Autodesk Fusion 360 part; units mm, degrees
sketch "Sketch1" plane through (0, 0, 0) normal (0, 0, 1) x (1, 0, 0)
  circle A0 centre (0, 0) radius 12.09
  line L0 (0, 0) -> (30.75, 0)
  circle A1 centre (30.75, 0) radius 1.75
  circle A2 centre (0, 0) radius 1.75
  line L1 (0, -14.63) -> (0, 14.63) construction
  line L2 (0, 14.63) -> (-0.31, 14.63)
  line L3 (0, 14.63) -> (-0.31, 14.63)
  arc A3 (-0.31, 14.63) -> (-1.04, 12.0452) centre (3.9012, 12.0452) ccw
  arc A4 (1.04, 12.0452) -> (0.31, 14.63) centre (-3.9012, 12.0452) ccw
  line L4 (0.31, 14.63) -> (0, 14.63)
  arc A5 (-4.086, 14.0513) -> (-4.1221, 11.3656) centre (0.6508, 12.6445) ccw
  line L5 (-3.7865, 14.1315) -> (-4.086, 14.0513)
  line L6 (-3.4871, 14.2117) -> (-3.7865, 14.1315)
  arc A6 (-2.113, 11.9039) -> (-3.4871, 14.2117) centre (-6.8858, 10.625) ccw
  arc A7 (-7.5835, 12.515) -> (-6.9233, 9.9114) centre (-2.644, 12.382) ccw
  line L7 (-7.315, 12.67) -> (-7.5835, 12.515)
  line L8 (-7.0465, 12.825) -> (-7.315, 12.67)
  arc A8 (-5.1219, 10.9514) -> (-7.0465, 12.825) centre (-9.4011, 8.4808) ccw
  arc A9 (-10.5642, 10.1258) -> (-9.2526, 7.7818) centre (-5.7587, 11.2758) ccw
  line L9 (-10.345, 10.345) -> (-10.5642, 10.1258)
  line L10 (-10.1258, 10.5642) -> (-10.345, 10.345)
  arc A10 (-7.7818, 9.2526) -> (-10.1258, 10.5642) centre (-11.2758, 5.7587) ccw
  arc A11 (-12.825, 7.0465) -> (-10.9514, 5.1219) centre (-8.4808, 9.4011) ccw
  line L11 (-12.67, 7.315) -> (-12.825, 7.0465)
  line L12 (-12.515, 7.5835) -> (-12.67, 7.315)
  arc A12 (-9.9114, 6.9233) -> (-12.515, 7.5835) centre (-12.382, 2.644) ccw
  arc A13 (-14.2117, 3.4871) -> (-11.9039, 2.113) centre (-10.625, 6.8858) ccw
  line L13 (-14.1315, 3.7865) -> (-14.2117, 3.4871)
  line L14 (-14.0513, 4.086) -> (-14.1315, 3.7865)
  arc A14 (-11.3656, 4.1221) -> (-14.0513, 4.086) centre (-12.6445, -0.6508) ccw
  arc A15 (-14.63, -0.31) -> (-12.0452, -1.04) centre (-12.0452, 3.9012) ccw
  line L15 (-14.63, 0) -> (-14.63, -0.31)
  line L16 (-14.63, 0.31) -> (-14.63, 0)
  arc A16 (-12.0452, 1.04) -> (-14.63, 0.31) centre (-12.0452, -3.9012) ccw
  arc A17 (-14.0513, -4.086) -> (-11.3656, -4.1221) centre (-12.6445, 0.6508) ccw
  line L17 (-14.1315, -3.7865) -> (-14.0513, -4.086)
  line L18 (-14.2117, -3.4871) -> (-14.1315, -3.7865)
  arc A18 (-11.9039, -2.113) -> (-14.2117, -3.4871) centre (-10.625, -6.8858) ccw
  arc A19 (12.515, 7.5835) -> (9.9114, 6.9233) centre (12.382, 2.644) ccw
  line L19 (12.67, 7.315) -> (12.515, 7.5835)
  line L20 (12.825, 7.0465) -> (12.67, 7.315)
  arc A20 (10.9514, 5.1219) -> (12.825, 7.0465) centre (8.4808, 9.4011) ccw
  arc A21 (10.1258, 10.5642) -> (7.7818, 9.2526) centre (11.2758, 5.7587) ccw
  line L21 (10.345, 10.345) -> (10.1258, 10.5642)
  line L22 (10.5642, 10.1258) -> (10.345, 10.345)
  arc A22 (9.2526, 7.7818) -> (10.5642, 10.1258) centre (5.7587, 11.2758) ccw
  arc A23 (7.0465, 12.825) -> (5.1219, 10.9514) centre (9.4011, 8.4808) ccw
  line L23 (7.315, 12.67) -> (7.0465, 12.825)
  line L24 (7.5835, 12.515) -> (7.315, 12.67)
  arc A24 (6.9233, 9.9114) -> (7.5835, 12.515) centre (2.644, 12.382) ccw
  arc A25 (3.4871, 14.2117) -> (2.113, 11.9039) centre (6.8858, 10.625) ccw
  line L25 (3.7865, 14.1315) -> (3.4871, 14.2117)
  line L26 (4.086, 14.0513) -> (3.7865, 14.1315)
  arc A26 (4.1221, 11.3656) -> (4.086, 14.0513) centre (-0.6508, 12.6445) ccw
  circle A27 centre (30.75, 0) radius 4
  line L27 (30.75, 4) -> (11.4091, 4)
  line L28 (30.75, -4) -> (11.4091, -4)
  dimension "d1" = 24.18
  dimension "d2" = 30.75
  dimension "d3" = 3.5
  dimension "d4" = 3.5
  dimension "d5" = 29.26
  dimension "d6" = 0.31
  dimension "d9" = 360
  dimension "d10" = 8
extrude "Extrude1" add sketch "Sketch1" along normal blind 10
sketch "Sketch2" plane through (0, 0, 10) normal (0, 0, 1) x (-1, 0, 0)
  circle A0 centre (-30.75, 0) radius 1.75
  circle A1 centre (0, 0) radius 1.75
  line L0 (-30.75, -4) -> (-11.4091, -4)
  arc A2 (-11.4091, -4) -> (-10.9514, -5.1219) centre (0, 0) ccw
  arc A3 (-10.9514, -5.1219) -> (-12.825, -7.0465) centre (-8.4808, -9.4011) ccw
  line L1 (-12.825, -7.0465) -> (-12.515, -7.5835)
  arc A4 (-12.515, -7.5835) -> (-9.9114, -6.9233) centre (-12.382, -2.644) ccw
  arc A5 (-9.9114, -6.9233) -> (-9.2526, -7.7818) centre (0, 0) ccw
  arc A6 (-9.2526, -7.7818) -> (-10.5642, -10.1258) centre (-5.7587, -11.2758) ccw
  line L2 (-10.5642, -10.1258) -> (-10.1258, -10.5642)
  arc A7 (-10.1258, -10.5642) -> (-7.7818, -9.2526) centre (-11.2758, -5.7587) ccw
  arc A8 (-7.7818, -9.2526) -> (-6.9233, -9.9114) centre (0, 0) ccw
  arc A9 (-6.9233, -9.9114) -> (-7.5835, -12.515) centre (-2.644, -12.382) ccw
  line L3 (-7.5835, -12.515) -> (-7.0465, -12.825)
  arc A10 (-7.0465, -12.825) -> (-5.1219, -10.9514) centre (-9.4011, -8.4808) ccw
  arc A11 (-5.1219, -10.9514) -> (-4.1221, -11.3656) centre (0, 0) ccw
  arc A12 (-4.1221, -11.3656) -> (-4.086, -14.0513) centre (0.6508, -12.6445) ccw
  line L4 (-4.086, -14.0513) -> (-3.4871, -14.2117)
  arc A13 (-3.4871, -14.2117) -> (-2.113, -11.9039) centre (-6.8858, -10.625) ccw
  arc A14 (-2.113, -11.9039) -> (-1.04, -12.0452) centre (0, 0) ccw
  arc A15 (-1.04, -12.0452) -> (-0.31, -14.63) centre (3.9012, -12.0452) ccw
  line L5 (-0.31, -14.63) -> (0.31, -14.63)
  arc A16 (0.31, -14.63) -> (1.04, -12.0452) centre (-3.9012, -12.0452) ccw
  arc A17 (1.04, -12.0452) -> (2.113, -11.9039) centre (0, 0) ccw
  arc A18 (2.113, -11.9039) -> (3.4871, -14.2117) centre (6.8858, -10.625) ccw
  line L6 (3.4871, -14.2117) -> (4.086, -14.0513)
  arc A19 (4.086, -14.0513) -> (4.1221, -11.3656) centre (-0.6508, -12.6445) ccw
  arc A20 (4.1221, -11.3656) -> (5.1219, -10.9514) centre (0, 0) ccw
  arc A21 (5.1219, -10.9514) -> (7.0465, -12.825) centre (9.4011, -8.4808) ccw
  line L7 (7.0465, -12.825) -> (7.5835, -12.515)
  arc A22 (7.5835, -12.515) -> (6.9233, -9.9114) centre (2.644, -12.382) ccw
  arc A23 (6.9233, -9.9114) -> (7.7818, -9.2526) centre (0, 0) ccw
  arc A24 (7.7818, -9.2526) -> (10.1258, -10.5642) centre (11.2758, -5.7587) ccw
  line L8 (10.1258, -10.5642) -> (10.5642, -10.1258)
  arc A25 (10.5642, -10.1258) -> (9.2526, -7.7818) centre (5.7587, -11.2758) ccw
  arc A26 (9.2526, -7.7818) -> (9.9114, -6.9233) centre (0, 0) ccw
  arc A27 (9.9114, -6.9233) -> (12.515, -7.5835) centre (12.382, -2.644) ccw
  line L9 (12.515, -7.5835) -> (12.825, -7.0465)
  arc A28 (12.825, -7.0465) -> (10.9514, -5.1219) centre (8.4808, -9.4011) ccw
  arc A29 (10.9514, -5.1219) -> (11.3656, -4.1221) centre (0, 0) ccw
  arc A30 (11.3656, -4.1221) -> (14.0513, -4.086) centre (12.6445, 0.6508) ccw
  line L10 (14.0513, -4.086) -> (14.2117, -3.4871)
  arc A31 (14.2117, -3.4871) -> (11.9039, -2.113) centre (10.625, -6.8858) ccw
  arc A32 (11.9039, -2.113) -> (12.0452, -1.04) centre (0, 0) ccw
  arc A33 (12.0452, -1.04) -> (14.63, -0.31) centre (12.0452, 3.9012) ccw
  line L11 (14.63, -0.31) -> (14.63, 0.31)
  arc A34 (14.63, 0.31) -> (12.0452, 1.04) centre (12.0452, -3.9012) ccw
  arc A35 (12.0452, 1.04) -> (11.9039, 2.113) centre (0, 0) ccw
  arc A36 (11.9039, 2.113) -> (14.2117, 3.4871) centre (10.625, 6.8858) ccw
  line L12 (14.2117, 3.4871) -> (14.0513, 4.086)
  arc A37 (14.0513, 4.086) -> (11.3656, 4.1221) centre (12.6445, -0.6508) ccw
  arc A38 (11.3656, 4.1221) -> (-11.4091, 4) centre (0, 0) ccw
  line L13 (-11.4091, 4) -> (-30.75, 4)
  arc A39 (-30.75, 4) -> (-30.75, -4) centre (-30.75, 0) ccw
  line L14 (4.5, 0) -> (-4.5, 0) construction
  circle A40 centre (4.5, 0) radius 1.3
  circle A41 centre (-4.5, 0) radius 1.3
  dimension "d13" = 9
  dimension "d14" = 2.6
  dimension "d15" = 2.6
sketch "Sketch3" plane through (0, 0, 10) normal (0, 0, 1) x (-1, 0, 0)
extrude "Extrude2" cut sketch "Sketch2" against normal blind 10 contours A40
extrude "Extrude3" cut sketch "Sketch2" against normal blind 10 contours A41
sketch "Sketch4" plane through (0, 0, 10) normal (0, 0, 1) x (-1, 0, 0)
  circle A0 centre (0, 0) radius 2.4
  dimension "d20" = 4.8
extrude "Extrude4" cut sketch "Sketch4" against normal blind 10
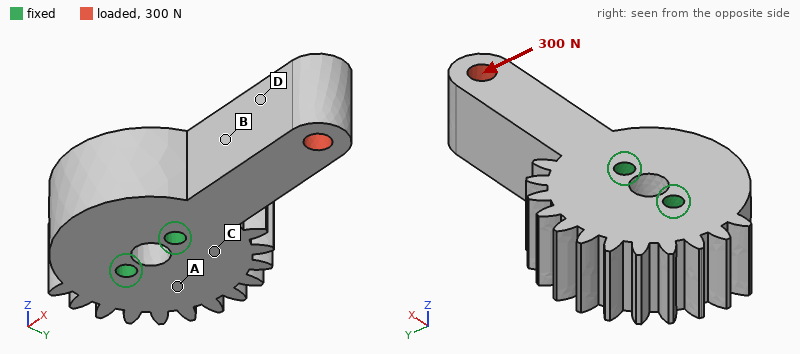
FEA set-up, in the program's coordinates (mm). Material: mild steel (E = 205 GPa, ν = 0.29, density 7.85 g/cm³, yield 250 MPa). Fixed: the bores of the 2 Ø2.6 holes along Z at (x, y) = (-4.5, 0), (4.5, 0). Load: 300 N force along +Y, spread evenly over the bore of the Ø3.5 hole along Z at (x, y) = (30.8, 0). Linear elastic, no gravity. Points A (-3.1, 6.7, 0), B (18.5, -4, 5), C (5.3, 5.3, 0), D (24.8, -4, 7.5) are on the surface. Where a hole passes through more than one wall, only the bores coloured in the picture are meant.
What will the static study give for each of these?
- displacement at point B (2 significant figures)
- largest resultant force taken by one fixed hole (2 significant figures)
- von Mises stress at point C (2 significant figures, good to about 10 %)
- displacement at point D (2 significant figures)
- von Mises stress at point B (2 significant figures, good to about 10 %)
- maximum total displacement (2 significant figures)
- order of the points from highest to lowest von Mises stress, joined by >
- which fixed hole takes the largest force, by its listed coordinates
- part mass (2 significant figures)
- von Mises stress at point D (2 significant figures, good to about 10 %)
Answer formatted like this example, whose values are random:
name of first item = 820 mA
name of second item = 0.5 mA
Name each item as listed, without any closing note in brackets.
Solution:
displacement at point B = 5.6 µm
largest resultant force taken by one fixed hole = 860 N
von Mises stress at point C = 12 MPa
displacement at point D = 11 µm
von Mises stress at point B = 35 MPa
maximum total displacement = 20 µm
order of the points from highest to lowest von Mises stress, joined by > = B > D > C > A
which fixed hole takes the largest force, by its listed coordinates = (4.5, 0)
part mass = 51 g
von Mises stress at point D = 17 MPa
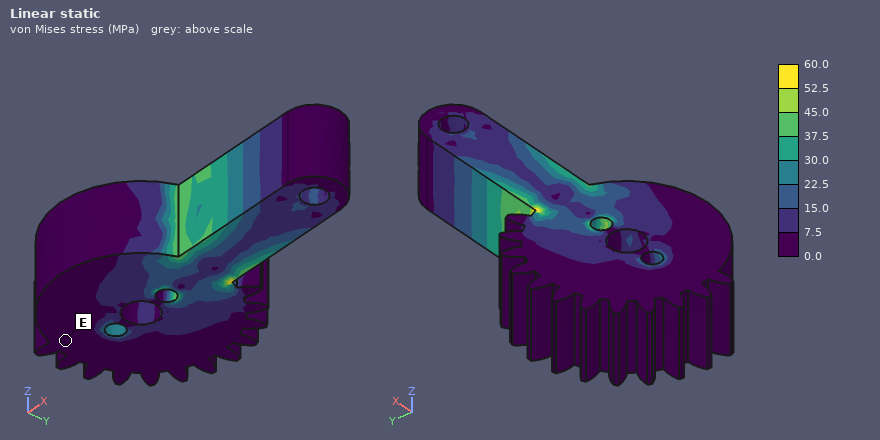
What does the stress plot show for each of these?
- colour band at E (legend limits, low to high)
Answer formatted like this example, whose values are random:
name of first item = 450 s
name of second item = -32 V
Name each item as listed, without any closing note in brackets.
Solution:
colour band at E = 0.0 to 7.5 MPa
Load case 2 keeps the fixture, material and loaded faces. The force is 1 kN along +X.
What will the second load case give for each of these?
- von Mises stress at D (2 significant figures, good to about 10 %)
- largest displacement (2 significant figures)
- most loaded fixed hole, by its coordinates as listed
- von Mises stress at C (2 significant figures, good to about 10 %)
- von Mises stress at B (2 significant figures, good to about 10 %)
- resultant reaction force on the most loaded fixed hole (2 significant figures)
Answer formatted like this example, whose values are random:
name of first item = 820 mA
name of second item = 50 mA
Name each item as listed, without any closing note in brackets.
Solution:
von Mises stress at D = 14 MPa
largest displacement = 2.0 µm
most loaded fixed hole, by its coordinates as listed = (4.5, 0)
von Mises stress at C = 3.6 MPa
von Mises stress at B = 13 MPa
resultant reaction force on the most loaded fixed hole = 820 N
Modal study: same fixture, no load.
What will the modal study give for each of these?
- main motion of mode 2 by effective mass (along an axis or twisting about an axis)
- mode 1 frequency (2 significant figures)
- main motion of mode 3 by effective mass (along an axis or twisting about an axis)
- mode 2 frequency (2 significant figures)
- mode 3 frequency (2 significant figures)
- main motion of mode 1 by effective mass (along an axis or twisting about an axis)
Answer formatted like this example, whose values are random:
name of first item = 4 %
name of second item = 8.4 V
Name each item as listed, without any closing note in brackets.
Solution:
main motion of mode 2 by effective mass = along Z
mode 1 frequency = 9300 Hz
main motion of mode 3 by effective mass = twisting about X
mode 2 frequency = 10 kHz
mode 3 frequency = 28 kHz
main motion of mode 1 by effective mass = along Y
